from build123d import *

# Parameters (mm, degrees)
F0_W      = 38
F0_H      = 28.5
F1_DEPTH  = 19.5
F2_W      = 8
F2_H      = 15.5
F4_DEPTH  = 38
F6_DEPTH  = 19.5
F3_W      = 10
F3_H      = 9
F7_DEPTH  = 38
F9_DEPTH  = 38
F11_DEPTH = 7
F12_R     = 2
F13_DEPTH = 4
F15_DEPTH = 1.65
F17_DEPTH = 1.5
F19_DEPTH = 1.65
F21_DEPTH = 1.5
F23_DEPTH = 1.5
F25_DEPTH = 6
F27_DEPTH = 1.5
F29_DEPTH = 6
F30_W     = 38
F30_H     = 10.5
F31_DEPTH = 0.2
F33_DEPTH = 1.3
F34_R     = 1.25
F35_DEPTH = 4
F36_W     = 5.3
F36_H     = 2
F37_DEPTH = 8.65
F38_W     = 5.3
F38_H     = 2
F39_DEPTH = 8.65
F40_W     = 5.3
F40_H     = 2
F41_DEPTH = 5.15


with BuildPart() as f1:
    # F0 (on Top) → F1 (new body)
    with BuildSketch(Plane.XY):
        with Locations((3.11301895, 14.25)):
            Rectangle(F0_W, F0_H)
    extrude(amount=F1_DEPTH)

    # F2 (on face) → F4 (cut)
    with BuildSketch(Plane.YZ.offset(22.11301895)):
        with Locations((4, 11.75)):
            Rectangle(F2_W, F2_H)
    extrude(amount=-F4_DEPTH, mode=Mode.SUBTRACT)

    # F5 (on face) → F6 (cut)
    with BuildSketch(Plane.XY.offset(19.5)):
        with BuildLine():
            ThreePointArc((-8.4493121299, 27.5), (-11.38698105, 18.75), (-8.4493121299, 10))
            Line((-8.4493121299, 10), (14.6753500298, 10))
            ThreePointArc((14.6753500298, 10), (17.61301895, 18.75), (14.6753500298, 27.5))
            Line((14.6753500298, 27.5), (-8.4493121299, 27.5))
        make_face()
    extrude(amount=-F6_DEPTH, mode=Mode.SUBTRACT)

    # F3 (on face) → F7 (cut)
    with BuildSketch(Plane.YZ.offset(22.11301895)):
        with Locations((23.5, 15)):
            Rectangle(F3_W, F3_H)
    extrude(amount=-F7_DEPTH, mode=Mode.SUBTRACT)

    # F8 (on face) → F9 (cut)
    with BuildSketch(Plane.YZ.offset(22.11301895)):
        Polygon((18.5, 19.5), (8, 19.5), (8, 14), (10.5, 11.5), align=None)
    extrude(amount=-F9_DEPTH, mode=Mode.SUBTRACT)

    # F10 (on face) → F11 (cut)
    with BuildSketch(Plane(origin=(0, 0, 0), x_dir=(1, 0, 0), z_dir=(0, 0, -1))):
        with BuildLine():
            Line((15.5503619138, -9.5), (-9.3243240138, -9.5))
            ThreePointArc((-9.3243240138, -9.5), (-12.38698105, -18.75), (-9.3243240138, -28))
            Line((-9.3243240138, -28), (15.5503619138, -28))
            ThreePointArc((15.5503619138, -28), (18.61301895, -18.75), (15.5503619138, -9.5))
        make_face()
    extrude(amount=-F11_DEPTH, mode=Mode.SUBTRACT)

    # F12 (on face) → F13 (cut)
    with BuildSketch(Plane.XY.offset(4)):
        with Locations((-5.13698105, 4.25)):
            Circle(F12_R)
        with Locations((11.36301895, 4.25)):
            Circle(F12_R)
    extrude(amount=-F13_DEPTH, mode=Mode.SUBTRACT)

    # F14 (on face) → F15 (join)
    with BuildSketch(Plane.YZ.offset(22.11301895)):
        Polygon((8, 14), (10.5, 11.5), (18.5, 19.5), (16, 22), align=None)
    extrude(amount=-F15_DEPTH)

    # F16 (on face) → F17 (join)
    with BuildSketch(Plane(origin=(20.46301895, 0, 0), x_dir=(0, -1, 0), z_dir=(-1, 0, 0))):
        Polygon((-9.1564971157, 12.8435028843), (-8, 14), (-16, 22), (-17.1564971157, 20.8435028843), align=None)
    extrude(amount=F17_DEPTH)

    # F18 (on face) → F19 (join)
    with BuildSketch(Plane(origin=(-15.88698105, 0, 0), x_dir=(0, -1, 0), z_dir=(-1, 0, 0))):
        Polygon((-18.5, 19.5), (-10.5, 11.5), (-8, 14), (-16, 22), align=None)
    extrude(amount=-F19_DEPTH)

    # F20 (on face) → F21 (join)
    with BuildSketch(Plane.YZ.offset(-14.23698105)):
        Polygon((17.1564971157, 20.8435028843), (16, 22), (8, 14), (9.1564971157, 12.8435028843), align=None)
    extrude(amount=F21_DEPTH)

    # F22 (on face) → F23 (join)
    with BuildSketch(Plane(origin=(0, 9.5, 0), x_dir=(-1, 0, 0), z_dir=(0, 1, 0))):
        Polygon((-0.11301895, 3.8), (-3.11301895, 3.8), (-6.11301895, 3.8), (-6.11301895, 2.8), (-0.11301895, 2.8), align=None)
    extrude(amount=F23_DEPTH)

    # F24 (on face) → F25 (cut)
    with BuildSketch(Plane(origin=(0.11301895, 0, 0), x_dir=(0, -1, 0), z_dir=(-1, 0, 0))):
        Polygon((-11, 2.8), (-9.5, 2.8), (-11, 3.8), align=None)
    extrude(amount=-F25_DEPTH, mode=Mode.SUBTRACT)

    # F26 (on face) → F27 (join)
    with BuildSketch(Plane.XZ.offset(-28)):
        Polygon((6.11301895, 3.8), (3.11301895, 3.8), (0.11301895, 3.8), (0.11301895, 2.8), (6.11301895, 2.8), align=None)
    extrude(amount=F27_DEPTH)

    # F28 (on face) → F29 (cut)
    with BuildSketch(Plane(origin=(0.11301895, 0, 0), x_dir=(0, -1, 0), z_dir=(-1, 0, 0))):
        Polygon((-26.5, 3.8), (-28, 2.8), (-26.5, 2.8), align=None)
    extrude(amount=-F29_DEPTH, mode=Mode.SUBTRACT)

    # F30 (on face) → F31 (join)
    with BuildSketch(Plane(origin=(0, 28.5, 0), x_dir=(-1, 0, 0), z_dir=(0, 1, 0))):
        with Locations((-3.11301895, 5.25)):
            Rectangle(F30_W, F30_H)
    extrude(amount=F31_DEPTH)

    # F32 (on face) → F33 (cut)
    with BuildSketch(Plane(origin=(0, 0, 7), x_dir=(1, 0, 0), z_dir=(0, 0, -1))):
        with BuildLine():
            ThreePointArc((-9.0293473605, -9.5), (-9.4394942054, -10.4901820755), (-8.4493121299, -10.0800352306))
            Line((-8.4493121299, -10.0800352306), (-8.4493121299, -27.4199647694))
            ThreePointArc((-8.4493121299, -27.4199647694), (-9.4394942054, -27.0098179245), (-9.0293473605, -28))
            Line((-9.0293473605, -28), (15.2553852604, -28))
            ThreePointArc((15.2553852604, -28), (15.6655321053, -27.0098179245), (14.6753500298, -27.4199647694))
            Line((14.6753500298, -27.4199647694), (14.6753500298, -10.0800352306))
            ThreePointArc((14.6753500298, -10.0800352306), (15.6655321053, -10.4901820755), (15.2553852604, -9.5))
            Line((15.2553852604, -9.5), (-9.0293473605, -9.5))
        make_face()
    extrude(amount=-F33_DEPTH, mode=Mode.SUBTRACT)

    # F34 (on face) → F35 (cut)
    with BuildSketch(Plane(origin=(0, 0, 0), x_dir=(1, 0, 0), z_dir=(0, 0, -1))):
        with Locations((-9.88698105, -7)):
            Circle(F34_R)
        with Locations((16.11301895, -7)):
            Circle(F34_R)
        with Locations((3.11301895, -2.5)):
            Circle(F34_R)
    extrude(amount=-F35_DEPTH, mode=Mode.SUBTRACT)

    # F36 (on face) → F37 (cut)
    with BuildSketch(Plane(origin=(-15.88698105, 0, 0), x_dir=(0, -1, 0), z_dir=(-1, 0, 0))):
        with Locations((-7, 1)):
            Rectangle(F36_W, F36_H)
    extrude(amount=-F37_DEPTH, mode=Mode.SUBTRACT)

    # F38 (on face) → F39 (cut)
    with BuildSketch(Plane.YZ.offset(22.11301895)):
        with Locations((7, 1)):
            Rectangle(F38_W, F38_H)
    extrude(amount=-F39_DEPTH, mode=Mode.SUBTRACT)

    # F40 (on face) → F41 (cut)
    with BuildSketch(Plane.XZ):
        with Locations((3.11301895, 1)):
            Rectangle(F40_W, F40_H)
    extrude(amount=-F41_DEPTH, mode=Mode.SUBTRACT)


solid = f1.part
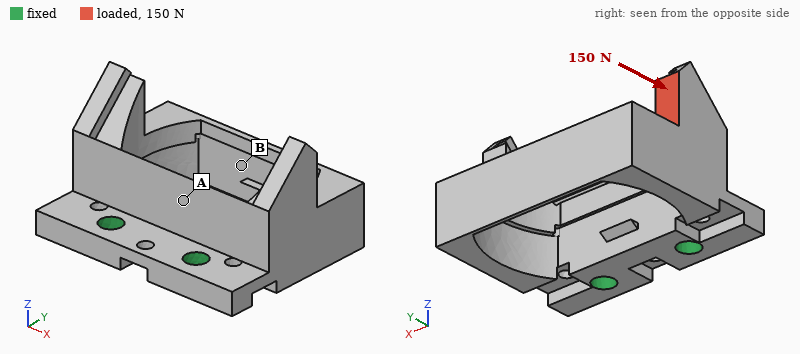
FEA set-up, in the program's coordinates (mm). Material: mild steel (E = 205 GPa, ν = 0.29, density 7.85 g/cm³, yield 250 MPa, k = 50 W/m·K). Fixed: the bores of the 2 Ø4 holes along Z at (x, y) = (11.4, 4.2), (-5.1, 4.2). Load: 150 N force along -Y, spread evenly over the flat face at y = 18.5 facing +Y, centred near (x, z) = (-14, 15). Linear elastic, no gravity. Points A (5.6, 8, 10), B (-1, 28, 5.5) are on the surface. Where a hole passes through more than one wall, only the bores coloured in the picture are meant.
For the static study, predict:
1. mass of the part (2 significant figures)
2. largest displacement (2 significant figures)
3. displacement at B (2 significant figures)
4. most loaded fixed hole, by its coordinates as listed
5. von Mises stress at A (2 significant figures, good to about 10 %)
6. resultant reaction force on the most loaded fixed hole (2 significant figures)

35 g
56 µm
42 µm
(-5.1, 4.2)
23 MPa
170 N
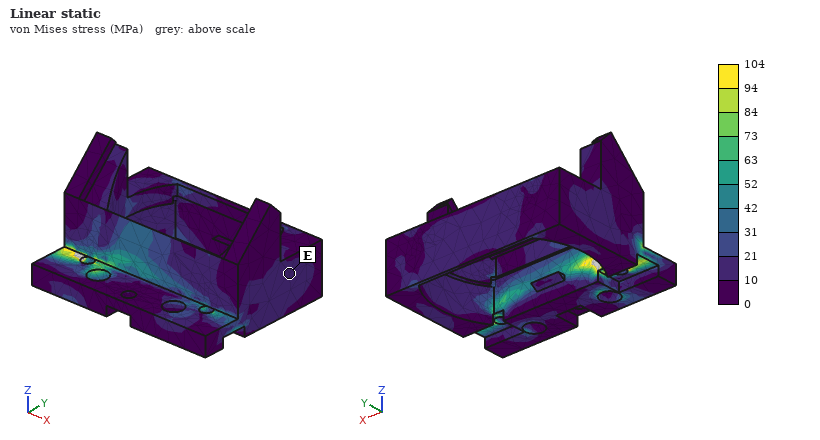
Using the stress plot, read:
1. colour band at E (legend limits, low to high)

10 to 21 MPa
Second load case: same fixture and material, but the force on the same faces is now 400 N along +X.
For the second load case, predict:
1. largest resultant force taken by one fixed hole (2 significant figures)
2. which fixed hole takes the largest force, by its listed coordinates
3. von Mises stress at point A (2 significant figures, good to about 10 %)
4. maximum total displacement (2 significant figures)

400 N
(11.4, 4.2)
39 MPa
37 µm
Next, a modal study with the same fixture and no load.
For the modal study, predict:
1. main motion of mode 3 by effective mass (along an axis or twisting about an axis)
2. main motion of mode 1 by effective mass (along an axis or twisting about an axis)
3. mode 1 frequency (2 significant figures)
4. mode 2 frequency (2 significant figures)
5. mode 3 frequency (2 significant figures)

along X
along Z
2300 Hz
3900 Hz
4900 Hz
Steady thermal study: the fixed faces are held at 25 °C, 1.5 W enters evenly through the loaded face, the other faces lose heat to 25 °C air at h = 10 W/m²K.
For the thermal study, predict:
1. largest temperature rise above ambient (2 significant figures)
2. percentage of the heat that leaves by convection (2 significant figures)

18 K
11 %
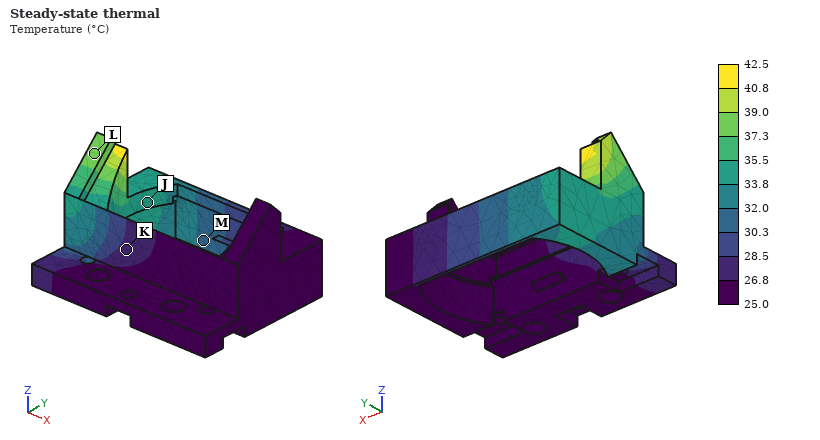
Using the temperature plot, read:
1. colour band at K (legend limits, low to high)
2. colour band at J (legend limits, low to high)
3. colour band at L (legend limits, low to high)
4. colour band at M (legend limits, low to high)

26.8 to 28.5 °C
33.8 to 35.5 °C
37.3 to 39.0 °C
30.3 to 32.0 °C
